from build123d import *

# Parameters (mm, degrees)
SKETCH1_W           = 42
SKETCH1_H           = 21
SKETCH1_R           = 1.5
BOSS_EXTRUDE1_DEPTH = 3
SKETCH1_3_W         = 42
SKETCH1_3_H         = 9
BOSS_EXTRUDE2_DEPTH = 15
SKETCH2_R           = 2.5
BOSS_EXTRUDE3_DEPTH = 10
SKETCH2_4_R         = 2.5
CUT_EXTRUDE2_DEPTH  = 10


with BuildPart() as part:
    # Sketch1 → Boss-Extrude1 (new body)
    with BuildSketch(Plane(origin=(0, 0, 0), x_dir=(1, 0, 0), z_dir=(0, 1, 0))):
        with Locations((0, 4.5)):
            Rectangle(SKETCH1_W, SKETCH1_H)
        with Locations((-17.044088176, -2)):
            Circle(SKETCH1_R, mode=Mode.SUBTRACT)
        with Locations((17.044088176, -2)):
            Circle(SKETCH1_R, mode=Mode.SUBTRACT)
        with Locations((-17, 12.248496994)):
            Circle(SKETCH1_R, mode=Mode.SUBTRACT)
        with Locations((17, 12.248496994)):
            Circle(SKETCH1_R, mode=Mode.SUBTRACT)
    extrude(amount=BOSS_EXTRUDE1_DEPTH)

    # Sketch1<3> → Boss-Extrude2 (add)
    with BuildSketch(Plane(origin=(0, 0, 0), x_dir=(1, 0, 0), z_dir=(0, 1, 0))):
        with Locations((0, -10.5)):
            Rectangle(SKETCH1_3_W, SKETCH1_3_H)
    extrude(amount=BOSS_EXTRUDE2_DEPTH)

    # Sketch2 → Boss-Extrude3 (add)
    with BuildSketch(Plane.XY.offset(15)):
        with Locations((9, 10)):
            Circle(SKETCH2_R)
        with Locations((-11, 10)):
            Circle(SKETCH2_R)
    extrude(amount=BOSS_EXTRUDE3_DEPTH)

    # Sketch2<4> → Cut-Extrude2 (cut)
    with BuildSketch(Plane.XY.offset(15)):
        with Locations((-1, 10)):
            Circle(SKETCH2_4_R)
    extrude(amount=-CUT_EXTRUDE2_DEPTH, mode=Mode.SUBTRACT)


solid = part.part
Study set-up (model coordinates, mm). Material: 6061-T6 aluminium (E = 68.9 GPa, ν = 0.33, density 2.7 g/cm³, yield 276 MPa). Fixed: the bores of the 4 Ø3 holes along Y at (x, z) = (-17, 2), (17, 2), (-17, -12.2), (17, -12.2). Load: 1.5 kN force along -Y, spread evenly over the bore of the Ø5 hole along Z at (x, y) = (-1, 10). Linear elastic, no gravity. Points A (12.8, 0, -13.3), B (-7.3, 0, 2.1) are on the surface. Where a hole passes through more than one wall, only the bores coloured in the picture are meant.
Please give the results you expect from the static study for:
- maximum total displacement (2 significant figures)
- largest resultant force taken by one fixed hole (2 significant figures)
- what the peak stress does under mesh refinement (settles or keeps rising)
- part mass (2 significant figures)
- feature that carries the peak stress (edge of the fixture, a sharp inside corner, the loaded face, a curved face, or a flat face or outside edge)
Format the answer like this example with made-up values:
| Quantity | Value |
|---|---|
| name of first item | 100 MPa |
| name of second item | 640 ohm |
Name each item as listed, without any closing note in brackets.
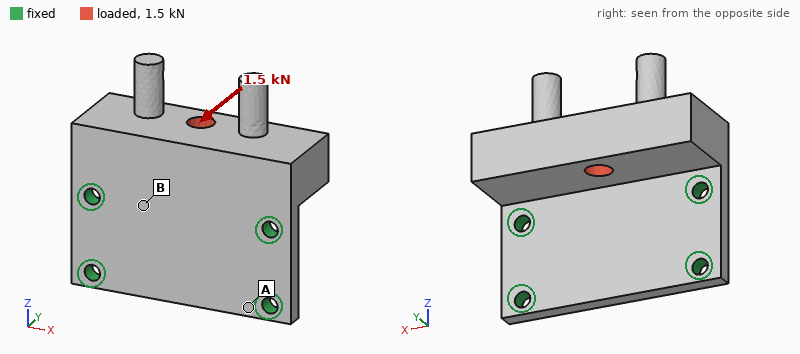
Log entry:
| Quantity | Value |
|---|---|
| maximum total displacement | 0.21 mm |
| largest resultant force taken by one fixed hole | 970 N |
| what the peak stress does under mesh refinement | keeps rising |
| part mass | 23 g |
| feature that carries the peak stress | edge of the fixture |
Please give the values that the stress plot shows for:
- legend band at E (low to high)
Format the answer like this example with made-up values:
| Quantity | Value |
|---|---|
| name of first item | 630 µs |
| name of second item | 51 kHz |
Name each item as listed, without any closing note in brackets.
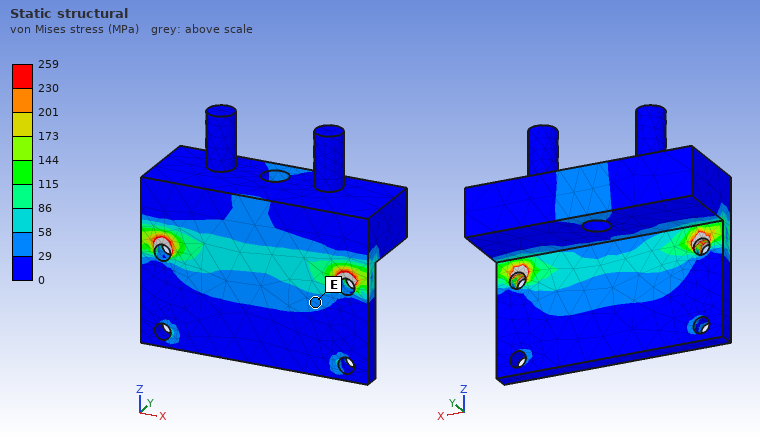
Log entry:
| Quantity | Value |
|---|---|
| legend band at E | 29 to 58 MPa |
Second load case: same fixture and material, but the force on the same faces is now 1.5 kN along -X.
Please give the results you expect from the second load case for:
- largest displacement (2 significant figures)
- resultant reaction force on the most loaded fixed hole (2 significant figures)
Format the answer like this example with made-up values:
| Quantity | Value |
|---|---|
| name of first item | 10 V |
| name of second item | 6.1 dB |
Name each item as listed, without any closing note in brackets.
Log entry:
| Quantity | Value |
|---|---|
| largest displacement | 16 µm |
| resultant reaction force on the most loaded fixed hole | 830 N |
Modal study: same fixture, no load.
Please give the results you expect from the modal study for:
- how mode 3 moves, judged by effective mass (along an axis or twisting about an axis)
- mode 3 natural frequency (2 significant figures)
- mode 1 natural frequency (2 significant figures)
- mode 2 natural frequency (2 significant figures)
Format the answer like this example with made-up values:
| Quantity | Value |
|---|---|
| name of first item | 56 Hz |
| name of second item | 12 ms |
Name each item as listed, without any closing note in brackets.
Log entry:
| Quantity | Value |
|---|---|
| how mode 3 moves, judged by effective mass | along Y |
| mode 3 natural frequency | 15 kHz |
| mode 1 natural frequency | 3800 Hz |
| mode 2 natural frequency | 12 kHz |
